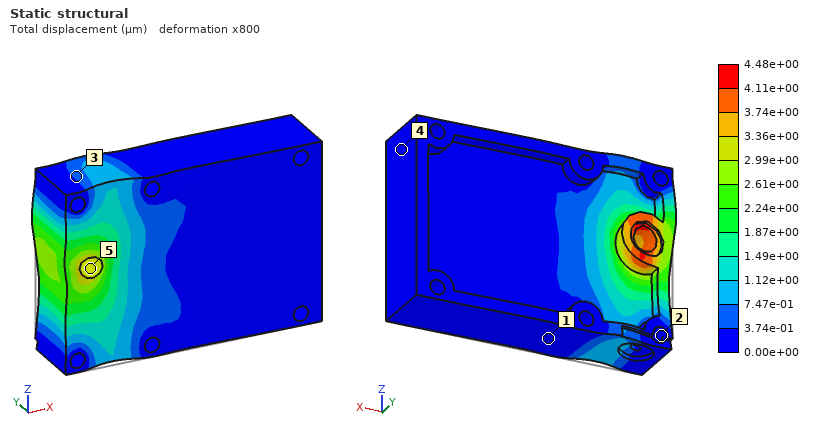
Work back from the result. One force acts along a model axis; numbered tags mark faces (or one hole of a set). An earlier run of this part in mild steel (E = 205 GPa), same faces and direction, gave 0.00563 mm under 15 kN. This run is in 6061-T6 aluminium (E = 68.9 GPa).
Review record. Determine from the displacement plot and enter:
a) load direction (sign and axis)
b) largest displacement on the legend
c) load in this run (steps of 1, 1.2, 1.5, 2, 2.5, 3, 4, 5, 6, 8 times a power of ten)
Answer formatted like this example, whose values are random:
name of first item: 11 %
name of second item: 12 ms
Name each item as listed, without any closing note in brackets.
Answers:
load direction: +Z
largest displacement on the legend: 4.48e+00 µm
load in this run: 4 kN
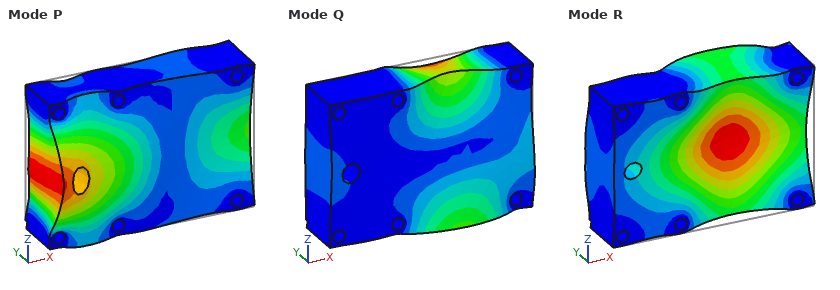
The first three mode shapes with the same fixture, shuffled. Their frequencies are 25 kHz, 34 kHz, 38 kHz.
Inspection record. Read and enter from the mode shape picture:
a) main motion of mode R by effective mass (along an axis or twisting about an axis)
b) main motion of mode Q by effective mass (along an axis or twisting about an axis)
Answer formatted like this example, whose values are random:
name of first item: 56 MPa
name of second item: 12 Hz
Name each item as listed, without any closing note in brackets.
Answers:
main motion of mode R by effective mass: along Y
main motion of mode Q by effective mass: along Z
